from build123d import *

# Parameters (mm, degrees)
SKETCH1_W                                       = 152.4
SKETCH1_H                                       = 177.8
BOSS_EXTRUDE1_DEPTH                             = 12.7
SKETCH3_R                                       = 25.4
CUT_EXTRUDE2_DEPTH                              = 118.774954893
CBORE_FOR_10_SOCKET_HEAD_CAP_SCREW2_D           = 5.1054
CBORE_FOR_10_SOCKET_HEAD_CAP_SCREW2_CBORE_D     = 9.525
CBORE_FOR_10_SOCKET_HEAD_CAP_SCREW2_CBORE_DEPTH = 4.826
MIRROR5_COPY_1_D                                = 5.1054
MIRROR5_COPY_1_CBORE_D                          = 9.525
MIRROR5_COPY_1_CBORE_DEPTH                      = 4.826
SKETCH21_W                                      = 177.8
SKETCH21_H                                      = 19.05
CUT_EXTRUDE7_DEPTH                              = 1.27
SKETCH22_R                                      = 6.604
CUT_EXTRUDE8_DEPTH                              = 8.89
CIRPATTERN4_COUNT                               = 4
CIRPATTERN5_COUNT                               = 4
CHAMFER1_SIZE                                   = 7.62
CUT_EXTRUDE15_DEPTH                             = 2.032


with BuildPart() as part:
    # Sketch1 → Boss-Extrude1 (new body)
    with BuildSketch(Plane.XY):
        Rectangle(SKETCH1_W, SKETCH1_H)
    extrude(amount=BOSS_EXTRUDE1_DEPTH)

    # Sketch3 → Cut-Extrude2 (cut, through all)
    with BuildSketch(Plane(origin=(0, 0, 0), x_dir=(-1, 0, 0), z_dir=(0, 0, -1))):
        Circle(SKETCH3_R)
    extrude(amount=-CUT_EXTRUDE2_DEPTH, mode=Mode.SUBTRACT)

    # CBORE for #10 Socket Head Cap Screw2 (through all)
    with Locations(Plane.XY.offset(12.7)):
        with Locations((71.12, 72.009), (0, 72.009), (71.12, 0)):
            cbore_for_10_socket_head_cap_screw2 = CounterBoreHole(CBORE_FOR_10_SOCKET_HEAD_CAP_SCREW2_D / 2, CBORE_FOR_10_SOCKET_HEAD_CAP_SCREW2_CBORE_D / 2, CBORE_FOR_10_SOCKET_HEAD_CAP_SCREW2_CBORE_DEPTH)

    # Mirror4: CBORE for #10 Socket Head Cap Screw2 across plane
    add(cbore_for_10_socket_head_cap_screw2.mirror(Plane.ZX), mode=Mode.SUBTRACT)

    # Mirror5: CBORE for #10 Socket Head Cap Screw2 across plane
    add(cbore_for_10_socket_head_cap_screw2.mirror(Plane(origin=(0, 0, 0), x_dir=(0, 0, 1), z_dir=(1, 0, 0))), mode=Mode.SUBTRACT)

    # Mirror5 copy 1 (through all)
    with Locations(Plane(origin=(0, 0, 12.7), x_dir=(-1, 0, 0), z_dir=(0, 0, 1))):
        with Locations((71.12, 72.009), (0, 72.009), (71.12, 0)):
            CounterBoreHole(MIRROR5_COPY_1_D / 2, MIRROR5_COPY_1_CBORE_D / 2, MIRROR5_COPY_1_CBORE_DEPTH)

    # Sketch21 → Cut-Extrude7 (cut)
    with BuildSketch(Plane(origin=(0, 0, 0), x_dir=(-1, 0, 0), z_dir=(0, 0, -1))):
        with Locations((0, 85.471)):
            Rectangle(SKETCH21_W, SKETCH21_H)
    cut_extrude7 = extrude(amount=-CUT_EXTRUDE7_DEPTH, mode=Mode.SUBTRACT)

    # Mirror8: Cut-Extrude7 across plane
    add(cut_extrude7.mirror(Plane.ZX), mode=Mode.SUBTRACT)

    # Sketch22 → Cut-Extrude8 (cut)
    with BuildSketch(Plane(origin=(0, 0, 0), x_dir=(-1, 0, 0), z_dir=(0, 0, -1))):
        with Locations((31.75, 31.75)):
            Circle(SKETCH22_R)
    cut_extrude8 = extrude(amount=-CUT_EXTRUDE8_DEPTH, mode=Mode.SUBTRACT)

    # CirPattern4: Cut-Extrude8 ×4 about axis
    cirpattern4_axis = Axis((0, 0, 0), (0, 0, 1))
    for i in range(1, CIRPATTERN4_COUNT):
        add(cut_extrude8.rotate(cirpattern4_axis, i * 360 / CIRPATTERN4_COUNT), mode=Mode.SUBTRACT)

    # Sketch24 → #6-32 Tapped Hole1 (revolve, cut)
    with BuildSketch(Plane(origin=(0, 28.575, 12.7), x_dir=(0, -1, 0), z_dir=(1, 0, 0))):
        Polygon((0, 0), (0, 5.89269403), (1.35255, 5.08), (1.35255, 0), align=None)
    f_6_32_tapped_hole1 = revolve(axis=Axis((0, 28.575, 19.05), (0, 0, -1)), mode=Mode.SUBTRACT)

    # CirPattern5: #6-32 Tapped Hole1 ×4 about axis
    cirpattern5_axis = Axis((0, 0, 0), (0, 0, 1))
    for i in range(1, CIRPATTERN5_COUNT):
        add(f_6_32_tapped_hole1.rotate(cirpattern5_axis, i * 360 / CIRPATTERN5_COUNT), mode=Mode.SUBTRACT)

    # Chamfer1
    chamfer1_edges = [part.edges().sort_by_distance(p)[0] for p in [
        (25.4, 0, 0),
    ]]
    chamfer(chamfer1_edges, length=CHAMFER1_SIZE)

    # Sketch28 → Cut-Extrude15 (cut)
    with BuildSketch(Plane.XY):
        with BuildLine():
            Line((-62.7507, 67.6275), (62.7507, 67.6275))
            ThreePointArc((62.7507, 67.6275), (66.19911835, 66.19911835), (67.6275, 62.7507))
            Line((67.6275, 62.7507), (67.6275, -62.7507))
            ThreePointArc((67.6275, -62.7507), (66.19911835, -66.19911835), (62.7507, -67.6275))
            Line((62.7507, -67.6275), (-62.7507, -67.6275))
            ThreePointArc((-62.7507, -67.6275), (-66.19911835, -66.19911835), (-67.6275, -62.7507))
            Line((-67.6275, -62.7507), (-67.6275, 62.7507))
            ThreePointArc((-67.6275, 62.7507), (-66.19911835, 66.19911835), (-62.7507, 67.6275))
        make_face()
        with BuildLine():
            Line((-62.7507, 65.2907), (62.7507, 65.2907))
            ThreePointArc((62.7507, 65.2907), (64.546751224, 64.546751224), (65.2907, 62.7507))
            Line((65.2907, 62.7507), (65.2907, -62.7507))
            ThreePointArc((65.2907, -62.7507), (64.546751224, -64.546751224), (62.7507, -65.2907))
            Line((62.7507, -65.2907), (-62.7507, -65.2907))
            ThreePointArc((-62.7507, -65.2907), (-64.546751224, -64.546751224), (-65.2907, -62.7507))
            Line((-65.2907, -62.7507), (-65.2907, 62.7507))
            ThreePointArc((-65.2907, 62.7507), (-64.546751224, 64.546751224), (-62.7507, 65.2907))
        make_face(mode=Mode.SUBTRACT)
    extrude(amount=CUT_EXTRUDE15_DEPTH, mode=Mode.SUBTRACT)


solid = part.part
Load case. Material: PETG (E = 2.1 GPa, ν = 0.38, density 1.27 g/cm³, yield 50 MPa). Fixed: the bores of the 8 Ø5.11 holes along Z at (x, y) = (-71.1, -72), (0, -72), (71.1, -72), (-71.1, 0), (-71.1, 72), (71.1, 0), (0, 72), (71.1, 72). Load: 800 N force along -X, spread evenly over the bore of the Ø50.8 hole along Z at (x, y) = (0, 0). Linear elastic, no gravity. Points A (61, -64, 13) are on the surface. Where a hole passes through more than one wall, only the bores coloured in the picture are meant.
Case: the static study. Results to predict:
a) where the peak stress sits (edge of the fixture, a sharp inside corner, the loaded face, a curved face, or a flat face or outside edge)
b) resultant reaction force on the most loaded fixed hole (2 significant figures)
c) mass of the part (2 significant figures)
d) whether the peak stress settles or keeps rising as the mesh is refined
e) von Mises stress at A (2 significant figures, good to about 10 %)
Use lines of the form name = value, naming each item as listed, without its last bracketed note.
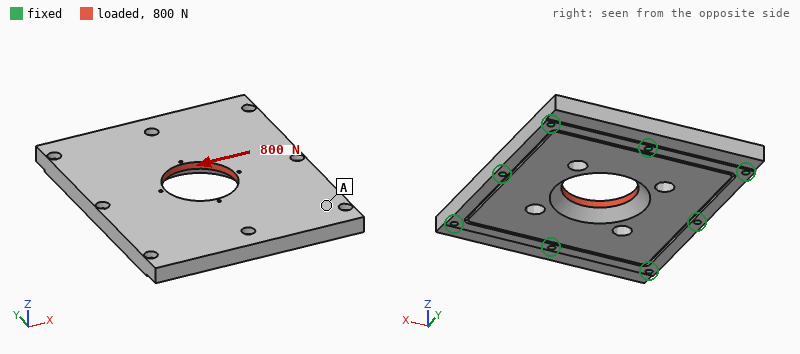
where the peak stress sits = edge of the fixture
resultant reaction force on the most loaded fixed hole = 170 N
mass of the part = 380 g
whether the peak stress settles or keeps rising as the mesh is refined = keeps rising
von Mises stress at A = 0.24 MPa
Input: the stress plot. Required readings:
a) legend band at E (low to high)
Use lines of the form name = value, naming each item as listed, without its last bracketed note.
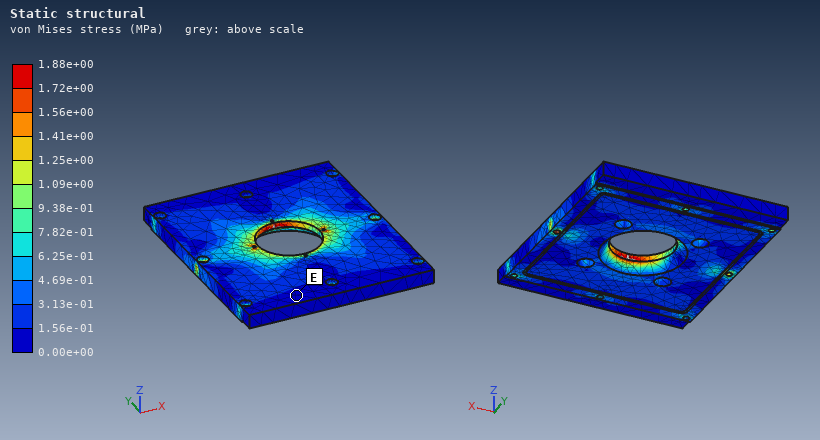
legend band at E = 0.00e+00 to 1.56e-01 MPa
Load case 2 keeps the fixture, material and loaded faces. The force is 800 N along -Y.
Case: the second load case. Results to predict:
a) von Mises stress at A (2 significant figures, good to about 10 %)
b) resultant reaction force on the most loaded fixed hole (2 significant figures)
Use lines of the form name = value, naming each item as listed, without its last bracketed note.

von Mises stress at A = 0.24 MPa
resultant reaction force on the most loaded fixed hole = 180 N
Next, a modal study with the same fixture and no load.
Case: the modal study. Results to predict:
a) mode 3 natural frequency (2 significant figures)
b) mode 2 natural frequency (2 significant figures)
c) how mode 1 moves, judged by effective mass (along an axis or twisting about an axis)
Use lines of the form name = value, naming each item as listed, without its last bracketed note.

mode 3 natural frequency = 1400 Hz
mode 2 natural frequency = 1400 Hz
how mode 1 moves, judged by effective mass = along Z
